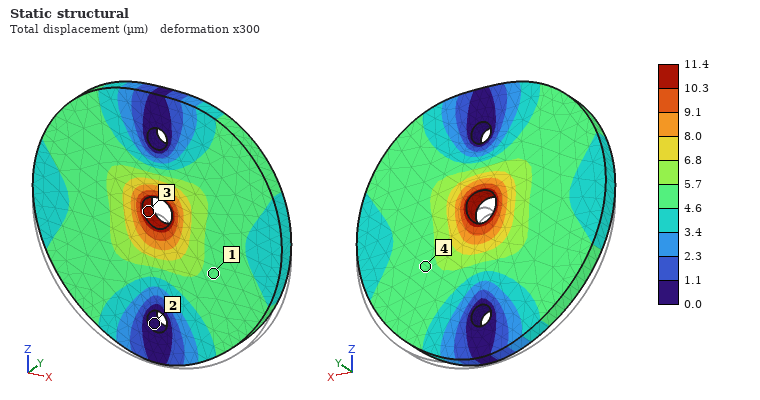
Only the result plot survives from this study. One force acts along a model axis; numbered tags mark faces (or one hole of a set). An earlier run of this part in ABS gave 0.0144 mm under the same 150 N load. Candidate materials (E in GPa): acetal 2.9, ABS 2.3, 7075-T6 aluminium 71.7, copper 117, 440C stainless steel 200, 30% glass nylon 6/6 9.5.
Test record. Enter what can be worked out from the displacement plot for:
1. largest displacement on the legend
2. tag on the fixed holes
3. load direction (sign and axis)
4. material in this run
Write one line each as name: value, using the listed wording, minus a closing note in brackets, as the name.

largest displacement on the legend: 11.4 µm
tag on the fixed holes: 2
load direction: +Z
material in this run: acetal
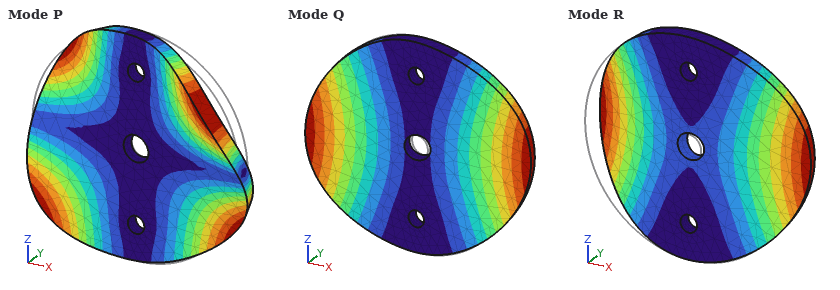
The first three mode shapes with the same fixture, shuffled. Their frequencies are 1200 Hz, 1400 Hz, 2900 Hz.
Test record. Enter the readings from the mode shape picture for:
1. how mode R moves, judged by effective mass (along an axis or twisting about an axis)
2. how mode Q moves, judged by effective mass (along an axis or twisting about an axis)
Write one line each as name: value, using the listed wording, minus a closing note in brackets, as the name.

how mode R moves, judged by effective mass: along Y
how mode Q moves, judged by effective mass: twisting about Z
